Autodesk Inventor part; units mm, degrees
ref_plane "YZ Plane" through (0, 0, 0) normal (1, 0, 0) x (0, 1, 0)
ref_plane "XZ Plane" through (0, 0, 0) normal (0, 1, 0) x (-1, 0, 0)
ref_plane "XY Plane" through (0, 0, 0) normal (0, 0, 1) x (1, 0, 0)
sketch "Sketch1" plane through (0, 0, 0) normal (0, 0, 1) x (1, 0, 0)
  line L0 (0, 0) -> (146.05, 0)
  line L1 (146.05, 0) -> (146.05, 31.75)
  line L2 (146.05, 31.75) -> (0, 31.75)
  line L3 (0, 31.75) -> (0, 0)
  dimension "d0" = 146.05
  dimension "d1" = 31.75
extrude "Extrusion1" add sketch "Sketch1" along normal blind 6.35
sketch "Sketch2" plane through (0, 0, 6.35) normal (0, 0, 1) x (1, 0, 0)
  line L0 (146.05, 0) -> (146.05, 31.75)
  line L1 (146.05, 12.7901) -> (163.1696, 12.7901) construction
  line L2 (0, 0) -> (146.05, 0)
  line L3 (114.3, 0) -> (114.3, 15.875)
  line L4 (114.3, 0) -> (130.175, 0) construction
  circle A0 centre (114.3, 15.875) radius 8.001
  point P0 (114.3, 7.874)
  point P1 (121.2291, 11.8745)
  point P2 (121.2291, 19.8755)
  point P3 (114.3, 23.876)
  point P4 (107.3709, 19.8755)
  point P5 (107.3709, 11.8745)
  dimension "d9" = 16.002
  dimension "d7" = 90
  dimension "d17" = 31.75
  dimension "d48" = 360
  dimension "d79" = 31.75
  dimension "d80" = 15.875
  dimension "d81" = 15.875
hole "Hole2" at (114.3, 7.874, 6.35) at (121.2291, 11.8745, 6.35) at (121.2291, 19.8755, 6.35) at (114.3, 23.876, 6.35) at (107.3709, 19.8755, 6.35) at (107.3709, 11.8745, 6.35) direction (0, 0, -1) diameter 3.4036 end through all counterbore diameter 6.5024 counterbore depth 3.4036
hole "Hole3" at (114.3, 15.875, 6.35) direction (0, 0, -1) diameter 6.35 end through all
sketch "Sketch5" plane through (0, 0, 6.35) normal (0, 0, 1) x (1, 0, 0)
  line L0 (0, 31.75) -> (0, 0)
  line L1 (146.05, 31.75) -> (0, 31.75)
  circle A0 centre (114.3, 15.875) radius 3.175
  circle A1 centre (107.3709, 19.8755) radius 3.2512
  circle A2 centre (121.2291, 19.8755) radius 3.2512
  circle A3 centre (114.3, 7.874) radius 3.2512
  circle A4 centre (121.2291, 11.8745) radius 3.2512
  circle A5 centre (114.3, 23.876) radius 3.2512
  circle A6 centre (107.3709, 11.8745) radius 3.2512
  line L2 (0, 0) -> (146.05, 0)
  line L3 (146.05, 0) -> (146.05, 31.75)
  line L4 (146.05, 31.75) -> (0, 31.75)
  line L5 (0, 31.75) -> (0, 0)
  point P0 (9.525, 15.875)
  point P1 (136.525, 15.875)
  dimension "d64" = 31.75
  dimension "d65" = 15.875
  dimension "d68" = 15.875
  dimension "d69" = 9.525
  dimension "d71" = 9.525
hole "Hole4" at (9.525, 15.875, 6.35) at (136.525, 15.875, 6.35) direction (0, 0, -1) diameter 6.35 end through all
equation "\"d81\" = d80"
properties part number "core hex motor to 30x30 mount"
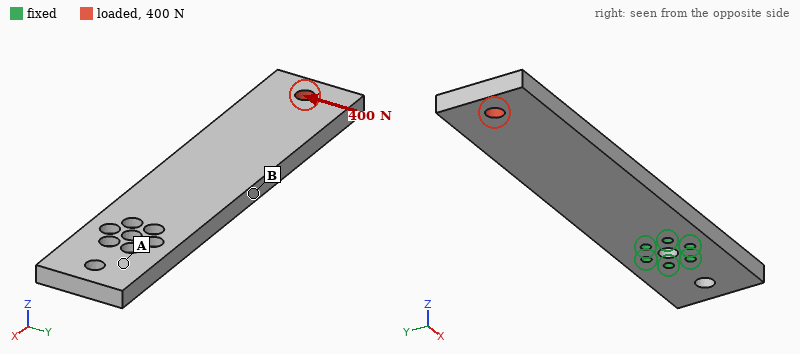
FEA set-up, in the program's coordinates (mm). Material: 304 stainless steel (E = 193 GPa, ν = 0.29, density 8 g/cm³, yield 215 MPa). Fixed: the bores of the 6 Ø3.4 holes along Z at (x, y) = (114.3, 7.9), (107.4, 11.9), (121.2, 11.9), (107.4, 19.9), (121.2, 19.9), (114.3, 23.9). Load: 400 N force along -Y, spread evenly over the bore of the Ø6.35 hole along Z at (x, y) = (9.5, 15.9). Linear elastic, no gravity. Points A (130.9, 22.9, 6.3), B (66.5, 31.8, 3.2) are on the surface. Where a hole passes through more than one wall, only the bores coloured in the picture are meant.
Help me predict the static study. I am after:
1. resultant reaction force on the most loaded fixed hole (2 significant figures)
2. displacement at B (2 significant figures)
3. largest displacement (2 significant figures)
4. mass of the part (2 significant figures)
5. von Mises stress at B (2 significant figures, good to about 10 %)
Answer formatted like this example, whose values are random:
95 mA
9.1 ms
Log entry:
1.0 kN
19 µm
65 µm
220 g
21 MPa
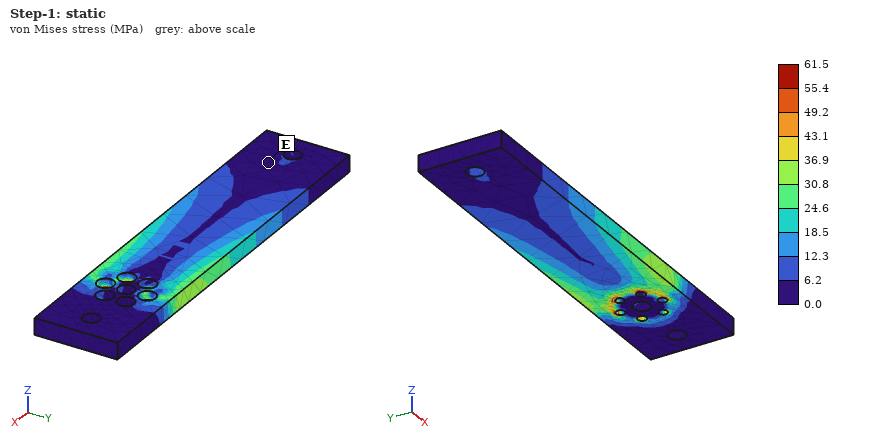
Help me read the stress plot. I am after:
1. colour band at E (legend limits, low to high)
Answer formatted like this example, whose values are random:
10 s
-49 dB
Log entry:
0.0 to 6.2 MPa
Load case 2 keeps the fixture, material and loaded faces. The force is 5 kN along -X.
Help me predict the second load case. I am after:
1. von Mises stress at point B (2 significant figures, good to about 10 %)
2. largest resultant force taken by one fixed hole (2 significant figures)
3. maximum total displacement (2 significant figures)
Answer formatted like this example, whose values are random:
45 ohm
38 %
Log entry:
25 MPa
1.4 kN
48 µm
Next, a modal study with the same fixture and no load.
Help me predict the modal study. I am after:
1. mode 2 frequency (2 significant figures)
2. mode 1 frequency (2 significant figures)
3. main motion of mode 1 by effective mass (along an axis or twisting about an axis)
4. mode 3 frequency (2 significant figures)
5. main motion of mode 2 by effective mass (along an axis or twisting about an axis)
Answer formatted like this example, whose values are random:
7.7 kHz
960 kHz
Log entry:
1700 Hz
400 Hz
along Z
2500 Hz
along Y
